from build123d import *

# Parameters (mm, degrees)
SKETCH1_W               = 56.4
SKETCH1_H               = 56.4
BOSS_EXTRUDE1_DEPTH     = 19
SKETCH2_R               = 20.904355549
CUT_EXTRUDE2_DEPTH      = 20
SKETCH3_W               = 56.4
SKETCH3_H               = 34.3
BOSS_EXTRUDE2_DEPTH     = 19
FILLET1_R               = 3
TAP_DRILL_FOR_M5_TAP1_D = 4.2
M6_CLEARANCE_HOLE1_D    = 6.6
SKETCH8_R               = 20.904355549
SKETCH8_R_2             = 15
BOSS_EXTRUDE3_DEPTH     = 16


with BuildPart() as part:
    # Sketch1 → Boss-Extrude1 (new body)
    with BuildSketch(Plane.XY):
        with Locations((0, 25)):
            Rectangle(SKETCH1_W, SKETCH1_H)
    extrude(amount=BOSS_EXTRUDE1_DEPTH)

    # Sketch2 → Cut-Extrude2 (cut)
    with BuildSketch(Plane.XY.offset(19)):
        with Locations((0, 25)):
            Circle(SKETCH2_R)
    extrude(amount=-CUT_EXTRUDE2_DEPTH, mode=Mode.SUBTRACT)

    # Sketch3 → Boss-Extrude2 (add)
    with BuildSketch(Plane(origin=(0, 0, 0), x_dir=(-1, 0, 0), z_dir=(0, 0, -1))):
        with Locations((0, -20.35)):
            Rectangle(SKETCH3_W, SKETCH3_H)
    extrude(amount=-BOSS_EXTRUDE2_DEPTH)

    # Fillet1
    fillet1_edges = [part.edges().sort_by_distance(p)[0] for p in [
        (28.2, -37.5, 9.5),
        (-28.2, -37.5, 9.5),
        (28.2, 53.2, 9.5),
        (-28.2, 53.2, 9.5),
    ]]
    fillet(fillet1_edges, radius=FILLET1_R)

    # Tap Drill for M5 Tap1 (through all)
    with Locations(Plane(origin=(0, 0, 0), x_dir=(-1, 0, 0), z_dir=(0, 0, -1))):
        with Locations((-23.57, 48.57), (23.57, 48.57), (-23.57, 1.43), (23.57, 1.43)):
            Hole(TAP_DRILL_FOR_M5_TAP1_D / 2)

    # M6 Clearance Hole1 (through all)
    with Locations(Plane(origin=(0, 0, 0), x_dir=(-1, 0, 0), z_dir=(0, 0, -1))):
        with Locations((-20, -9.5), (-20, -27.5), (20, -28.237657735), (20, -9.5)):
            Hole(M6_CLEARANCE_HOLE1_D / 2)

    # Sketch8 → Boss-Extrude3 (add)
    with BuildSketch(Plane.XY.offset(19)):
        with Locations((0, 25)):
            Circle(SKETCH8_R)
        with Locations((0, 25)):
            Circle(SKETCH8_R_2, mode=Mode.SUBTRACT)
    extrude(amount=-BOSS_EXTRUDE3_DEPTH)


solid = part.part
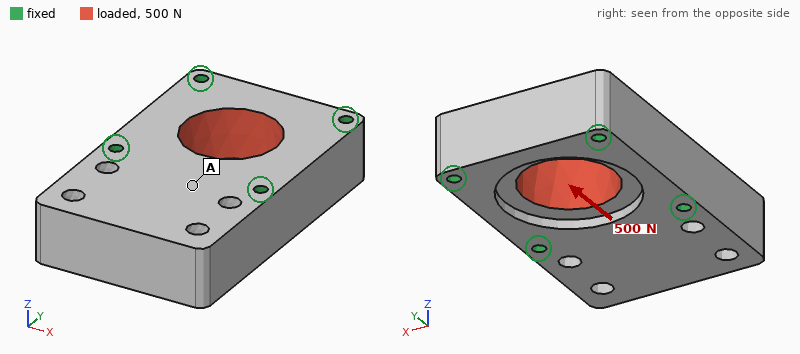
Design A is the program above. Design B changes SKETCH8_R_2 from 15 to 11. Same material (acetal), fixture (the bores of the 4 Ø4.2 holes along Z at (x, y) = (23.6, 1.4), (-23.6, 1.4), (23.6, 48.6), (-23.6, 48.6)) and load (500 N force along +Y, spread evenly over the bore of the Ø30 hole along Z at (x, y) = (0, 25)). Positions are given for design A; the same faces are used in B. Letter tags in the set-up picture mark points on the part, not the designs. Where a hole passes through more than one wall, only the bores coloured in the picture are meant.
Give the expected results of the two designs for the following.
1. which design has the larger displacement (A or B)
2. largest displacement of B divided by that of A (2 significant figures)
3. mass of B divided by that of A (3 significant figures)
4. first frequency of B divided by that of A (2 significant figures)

A
0.81
1.07
1.0
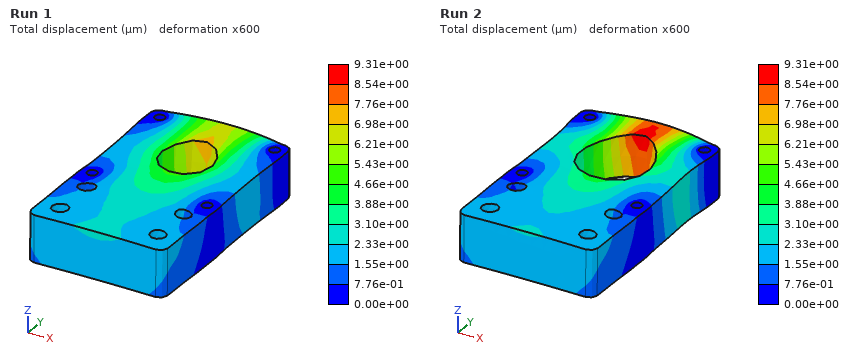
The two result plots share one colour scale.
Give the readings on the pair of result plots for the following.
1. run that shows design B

Run 1
